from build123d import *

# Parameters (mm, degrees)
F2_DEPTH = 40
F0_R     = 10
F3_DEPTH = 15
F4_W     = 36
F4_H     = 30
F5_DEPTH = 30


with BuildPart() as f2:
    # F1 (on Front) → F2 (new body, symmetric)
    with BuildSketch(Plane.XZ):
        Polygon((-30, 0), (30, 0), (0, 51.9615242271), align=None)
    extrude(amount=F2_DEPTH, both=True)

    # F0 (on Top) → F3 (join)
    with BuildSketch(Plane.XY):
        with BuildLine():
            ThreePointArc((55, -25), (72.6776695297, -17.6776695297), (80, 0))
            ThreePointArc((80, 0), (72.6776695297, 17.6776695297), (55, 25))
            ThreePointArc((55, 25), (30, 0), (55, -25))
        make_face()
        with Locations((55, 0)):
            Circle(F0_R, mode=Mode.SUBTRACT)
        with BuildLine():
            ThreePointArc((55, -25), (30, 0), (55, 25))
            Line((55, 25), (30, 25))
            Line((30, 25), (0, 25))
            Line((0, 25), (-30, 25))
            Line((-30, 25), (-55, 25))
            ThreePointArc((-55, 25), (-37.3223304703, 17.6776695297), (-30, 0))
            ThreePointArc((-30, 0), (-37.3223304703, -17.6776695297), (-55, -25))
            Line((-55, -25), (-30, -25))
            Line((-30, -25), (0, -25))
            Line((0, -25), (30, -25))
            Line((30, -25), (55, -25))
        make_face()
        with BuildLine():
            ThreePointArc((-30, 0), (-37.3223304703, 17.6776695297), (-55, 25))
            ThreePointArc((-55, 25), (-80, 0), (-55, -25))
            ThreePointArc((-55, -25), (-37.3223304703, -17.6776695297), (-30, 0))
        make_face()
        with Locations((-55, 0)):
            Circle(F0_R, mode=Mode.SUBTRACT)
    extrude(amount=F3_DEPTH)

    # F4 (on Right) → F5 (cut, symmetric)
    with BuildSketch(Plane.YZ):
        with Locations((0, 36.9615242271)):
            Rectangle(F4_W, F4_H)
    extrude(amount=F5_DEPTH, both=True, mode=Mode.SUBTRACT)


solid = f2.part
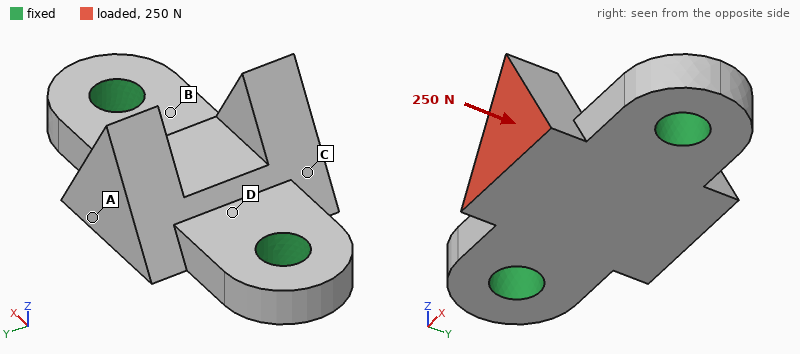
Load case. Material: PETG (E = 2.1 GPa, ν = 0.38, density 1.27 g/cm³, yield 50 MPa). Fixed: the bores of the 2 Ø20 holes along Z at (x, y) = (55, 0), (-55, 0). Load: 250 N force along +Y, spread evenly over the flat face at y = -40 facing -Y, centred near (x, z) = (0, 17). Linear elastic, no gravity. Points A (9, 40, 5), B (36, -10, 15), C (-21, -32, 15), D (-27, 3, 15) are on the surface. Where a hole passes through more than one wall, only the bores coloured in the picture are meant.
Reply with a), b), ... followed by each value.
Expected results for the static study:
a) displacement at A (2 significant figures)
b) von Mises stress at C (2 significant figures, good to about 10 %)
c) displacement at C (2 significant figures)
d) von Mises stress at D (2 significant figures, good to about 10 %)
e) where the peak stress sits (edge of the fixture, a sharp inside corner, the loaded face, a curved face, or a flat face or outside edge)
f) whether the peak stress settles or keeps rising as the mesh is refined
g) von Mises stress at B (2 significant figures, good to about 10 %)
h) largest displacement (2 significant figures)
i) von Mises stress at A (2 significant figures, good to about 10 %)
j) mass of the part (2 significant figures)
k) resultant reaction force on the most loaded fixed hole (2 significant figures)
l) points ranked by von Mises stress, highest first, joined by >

a) 30 µm
b) 0.44 MPa
c) 37 µm
d) 0.66 MPa
e) edge of the fixture
f) keeps rising
g) 0.86 MPa
h) 88 µm
i) 0.14 MPa
j) 220 g
k) 130 N
l) B > D > C > A
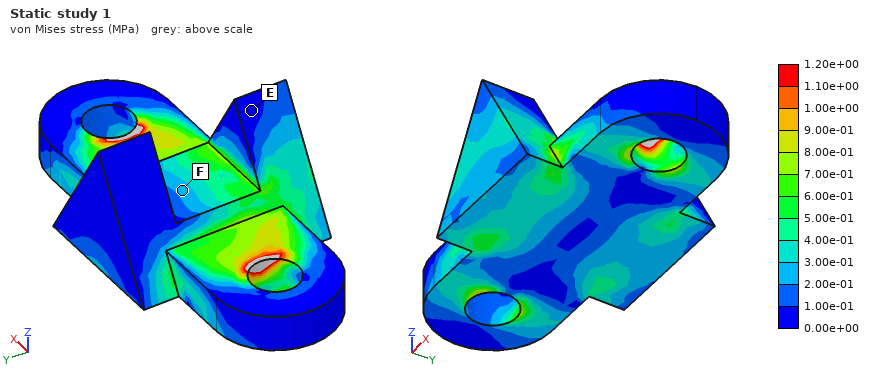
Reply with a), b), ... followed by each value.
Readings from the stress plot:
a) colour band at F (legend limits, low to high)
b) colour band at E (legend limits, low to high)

a) 2.00e-01 to 3.00e-01 MPa
b) 0.00e+00 to 1.00e-01 MPa
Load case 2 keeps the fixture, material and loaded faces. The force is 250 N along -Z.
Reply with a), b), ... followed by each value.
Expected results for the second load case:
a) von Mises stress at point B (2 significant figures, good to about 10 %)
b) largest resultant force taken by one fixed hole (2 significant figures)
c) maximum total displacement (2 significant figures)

a) 2.0 MPa
b) 140 N
c) 0.28 mm
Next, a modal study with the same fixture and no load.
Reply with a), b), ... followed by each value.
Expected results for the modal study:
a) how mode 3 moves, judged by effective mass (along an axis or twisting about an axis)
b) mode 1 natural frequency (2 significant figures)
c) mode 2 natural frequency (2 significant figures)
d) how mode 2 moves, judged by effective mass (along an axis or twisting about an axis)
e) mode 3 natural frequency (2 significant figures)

a) along Y
b) 840 Hz
c) 1200 Hz
d) along Z
e) 2200 Hz
